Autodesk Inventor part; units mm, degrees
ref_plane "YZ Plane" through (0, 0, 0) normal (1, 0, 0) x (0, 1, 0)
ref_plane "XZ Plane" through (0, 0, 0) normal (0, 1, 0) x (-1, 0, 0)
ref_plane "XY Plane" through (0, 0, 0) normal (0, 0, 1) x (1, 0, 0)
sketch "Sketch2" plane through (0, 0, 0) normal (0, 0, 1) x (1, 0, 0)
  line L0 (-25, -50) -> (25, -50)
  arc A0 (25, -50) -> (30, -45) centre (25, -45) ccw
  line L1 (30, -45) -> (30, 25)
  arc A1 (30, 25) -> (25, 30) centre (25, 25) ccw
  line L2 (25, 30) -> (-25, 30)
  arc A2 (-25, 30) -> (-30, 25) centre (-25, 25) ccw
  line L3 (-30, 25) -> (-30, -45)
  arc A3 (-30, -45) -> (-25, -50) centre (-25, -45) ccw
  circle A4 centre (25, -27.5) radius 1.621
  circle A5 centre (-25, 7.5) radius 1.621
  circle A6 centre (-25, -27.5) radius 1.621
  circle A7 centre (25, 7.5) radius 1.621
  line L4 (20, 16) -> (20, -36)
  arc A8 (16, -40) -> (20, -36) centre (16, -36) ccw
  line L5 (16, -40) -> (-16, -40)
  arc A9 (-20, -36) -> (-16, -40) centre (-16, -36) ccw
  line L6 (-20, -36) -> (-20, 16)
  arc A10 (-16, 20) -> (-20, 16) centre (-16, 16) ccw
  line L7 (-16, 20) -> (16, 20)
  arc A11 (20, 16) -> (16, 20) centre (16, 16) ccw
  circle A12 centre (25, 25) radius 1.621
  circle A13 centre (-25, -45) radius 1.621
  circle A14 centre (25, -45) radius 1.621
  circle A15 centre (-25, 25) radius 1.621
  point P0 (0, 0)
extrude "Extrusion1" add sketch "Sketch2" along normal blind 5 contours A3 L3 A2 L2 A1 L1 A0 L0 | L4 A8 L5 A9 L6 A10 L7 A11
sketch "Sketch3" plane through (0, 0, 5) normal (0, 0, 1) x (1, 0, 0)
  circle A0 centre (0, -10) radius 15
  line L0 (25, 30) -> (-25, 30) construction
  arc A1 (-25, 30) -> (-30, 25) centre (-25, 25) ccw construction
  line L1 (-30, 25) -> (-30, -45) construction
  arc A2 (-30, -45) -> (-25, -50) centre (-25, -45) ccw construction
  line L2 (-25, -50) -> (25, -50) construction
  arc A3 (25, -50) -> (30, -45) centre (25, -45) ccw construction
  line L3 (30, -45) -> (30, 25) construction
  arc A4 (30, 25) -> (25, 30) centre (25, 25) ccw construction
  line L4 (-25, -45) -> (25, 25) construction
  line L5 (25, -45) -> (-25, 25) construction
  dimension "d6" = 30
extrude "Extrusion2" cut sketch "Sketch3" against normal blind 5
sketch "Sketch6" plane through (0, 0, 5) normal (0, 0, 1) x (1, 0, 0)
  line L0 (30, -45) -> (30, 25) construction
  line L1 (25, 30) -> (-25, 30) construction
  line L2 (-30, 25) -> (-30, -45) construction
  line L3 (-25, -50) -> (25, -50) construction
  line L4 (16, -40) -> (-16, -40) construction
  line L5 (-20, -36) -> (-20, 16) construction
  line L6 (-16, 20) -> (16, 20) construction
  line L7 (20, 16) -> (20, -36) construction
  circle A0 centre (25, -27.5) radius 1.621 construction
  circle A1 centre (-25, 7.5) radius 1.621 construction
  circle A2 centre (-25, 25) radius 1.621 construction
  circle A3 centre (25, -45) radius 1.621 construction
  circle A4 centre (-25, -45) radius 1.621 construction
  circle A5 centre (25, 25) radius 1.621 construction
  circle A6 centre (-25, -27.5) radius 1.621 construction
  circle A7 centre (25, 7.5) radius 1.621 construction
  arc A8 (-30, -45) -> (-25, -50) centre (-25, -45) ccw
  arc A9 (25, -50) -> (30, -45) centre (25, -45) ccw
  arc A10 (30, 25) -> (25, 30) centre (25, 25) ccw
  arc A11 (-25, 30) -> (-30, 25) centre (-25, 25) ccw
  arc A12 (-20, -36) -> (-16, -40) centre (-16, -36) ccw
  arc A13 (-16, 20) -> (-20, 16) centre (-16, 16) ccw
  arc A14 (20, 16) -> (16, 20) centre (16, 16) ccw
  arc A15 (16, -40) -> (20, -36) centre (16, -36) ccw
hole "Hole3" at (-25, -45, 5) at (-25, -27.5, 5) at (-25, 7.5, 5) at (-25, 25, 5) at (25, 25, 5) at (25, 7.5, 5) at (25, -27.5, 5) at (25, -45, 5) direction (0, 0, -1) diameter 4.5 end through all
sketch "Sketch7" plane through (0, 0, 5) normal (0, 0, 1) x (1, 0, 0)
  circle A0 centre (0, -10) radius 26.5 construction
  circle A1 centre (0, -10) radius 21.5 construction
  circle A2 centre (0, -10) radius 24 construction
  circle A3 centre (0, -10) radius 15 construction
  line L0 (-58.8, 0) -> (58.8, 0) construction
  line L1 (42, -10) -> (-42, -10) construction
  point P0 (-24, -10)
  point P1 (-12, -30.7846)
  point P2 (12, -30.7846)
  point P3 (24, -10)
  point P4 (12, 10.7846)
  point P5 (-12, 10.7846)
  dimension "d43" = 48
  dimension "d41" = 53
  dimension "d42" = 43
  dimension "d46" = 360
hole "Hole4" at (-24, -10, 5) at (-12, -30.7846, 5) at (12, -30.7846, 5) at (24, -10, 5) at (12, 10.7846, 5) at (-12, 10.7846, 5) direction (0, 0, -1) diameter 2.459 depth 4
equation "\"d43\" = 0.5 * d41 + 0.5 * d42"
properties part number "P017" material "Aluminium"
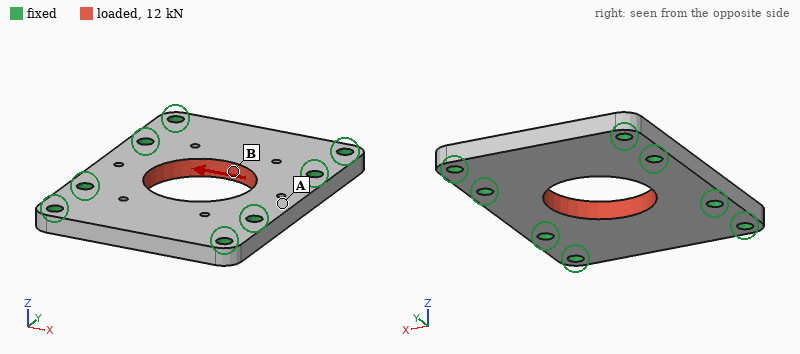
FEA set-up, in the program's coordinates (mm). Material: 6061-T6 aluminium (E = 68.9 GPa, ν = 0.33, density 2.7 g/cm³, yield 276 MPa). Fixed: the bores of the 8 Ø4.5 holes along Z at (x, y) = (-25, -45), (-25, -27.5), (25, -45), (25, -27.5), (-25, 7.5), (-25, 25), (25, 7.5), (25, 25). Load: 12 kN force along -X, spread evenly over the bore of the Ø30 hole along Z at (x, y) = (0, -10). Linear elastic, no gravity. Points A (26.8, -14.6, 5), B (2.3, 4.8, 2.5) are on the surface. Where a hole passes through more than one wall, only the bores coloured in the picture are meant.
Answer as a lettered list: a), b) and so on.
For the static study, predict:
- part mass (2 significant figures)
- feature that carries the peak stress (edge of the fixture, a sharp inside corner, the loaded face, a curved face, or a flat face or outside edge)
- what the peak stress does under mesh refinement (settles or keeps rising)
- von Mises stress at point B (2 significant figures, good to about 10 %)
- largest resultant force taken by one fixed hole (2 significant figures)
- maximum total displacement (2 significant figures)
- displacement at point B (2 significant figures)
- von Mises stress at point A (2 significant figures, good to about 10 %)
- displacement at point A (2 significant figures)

a) 53 g
b) edge of the fixture
c) keeps rising
d) 44 MPa
e) 2.6 kN
f) 15 µm
g) 9.0 µm
h) 15 MPa
i) 11 µm
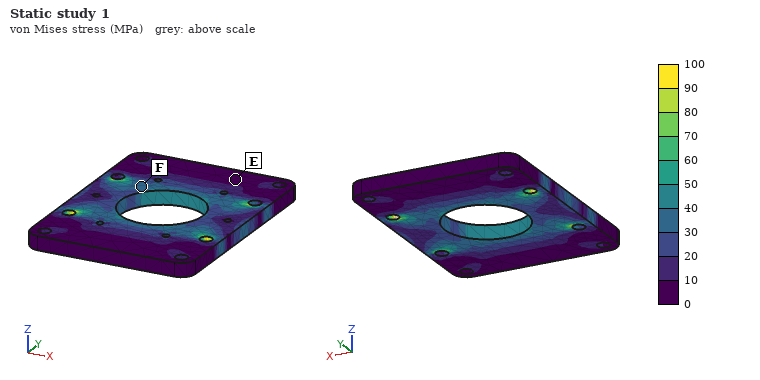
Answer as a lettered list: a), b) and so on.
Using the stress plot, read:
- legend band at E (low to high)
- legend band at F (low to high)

a) 0 to 10 MPa
b) 30 to 40 MPa
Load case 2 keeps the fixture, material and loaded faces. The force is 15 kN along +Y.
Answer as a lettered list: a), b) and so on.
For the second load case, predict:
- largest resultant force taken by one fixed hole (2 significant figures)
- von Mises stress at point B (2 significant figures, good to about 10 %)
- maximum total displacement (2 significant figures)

a) 2.6 kN
b) 32 MPa
c) 18 µm
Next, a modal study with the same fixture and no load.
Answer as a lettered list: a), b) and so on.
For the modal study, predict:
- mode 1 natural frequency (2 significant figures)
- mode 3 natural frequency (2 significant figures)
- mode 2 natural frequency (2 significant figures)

a) 11 kHz
b) 15 kHz
c) 11 kHz
